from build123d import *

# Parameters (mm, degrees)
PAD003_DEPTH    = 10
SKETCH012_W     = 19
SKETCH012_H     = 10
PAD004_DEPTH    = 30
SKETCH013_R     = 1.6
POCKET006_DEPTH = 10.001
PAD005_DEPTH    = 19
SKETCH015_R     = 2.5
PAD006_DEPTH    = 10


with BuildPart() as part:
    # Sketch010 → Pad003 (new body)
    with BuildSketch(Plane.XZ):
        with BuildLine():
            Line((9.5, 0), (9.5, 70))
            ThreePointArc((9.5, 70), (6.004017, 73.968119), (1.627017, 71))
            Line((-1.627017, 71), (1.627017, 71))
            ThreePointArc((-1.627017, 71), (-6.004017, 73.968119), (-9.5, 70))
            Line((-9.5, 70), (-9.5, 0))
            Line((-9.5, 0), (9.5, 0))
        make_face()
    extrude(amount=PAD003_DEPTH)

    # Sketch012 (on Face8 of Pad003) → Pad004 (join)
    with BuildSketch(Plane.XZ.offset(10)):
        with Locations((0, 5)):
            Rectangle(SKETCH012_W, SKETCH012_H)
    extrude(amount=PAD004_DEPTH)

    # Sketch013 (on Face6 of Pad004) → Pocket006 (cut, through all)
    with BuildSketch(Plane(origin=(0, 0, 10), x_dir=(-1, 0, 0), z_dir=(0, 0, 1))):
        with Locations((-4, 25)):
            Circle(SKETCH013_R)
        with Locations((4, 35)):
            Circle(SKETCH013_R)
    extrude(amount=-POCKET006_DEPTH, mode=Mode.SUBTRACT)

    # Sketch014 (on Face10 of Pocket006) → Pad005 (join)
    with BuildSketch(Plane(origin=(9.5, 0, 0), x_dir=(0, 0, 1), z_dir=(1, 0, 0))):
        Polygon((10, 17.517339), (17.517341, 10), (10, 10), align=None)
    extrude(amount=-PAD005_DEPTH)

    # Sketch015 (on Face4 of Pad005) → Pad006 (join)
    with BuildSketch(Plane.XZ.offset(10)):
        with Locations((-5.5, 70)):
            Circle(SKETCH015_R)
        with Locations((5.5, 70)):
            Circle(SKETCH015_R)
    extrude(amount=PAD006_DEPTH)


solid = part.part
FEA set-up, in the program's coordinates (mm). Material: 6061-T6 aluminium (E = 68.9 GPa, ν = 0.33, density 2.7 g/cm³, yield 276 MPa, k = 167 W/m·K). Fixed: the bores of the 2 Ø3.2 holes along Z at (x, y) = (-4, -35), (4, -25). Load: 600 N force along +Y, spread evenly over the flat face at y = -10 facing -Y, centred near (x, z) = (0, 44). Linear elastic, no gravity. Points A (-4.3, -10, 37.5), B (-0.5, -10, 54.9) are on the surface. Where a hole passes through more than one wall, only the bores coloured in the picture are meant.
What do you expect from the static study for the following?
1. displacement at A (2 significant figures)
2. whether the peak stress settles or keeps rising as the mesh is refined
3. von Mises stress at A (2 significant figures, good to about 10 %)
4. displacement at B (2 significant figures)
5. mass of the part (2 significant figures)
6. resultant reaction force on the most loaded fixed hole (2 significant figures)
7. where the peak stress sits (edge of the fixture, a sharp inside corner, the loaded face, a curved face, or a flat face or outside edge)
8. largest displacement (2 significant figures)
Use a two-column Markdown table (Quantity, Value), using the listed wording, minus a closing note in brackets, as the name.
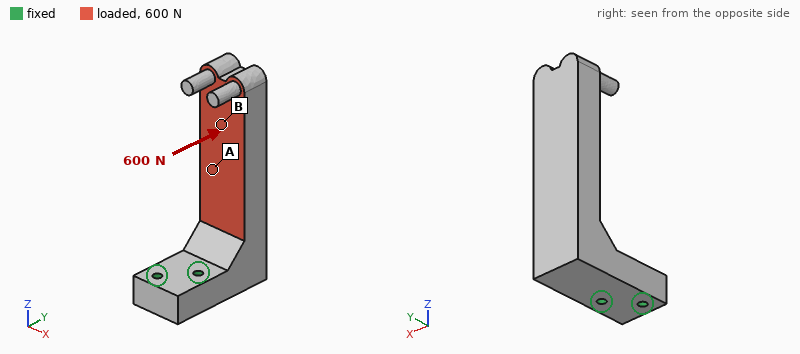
| Quantity | Value |
|---|---|
| displacement at A | 0.15 mm |
| whether the peak stress settles or keeps rising as the mesh is refined | keeps rising |
| von Mises stress at A | 20 MPa |
| displacement at B | 0.26 mm |
| mass of the part | 55 g |
| resultant reaction force on the most loaded fixed hole | 700 N |
| where the peak stress sits | edge of the fixture |
| largest displacement | 0.39 mm |
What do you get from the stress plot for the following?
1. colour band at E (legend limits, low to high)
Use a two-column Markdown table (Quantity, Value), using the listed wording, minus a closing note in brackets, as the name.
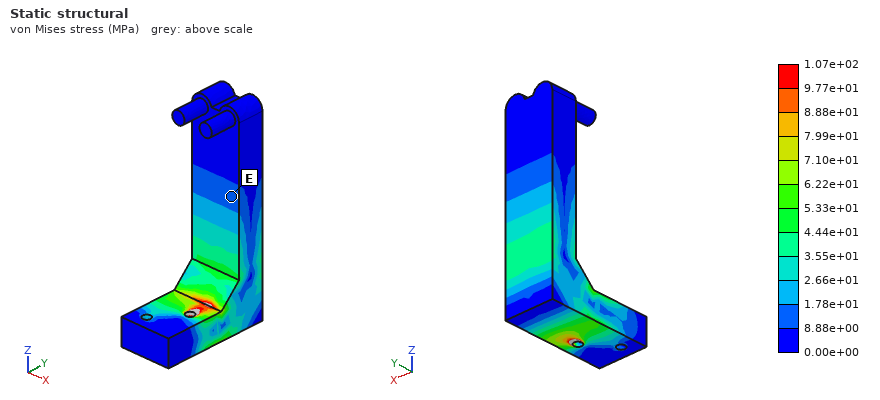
| Quantity | Value |
|---|---|
| colour band at E | 8.88e+00 to 1.78e+01 MPa |
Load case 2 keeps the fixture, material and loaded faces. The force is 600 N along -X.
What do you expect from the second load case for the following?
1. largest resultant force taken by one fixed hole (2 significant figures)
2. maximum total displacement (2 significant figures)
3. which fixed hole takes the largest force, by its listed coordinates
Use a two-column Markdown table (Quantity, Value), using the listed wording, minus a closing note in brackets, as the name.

| Quantity | Value |
|---|---|
| largest resultant force taken by one fixed hole | 1.2 kN |
| maximum total displacement | 0.27 mm |
| which fixed hole takes the largest force, by its listed coordinates | (4, -25) |
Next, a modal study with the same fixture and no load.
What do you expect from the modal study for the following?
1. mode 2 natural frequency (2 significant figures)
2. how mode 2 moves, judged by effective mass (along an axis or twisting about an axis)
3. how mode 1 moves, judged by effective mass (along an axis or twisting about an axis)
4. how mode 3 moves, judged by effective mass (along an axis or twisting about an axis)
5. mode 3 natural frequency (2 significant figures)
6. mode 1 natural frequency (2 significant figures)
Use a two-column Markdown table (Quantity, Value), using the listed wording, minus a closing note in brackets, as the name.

| Quantity | Value |
|---|---|
| mode 2 natural frequency | 1600 Hz |
| how mode 2 moves, judged by effective mass | along X |
| how mode 1 moves, judged by effective mass | along Y |
| how mode 3 moves, judged by effective mass | along Z |
| mode 3 natural frequency | 5300 Hz |
| mode 1 natural frequency | 1300 Hz |
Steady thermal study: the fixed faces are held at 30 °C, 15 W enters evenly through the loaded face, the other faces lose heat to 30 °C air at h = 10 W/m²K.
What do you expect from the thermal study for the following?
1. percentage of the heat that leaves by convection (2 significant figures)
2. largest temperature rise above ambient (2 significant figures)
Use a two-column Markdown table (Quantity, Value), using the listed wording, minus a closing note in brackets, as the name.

| Quantity | Value |
|---|---|
| percentage of the heat that leaves by convection | 4.4 % |
| largest temperature rise above ambient | 23 K |
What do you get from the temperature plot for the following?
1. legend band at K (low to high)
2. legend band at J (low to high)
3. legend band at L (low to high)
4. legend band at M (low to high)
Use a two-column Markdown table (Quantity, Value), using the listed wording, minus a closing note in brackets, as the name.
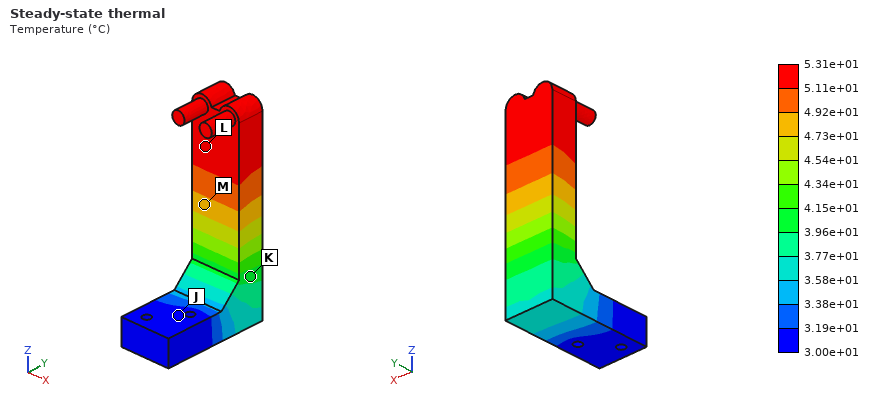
| Quantity | Value |
|---|---|
| legend band at K | 3.96e+01 to 4.15e+01 °C |
| legend band at J | 3.00e+01 to 3.19e+01 °C |
| legend band at L | 5.11e+01 to 5.31e+01 °C |
| legend band at M | 4.73e+01 to 4.92e+01 °C |
